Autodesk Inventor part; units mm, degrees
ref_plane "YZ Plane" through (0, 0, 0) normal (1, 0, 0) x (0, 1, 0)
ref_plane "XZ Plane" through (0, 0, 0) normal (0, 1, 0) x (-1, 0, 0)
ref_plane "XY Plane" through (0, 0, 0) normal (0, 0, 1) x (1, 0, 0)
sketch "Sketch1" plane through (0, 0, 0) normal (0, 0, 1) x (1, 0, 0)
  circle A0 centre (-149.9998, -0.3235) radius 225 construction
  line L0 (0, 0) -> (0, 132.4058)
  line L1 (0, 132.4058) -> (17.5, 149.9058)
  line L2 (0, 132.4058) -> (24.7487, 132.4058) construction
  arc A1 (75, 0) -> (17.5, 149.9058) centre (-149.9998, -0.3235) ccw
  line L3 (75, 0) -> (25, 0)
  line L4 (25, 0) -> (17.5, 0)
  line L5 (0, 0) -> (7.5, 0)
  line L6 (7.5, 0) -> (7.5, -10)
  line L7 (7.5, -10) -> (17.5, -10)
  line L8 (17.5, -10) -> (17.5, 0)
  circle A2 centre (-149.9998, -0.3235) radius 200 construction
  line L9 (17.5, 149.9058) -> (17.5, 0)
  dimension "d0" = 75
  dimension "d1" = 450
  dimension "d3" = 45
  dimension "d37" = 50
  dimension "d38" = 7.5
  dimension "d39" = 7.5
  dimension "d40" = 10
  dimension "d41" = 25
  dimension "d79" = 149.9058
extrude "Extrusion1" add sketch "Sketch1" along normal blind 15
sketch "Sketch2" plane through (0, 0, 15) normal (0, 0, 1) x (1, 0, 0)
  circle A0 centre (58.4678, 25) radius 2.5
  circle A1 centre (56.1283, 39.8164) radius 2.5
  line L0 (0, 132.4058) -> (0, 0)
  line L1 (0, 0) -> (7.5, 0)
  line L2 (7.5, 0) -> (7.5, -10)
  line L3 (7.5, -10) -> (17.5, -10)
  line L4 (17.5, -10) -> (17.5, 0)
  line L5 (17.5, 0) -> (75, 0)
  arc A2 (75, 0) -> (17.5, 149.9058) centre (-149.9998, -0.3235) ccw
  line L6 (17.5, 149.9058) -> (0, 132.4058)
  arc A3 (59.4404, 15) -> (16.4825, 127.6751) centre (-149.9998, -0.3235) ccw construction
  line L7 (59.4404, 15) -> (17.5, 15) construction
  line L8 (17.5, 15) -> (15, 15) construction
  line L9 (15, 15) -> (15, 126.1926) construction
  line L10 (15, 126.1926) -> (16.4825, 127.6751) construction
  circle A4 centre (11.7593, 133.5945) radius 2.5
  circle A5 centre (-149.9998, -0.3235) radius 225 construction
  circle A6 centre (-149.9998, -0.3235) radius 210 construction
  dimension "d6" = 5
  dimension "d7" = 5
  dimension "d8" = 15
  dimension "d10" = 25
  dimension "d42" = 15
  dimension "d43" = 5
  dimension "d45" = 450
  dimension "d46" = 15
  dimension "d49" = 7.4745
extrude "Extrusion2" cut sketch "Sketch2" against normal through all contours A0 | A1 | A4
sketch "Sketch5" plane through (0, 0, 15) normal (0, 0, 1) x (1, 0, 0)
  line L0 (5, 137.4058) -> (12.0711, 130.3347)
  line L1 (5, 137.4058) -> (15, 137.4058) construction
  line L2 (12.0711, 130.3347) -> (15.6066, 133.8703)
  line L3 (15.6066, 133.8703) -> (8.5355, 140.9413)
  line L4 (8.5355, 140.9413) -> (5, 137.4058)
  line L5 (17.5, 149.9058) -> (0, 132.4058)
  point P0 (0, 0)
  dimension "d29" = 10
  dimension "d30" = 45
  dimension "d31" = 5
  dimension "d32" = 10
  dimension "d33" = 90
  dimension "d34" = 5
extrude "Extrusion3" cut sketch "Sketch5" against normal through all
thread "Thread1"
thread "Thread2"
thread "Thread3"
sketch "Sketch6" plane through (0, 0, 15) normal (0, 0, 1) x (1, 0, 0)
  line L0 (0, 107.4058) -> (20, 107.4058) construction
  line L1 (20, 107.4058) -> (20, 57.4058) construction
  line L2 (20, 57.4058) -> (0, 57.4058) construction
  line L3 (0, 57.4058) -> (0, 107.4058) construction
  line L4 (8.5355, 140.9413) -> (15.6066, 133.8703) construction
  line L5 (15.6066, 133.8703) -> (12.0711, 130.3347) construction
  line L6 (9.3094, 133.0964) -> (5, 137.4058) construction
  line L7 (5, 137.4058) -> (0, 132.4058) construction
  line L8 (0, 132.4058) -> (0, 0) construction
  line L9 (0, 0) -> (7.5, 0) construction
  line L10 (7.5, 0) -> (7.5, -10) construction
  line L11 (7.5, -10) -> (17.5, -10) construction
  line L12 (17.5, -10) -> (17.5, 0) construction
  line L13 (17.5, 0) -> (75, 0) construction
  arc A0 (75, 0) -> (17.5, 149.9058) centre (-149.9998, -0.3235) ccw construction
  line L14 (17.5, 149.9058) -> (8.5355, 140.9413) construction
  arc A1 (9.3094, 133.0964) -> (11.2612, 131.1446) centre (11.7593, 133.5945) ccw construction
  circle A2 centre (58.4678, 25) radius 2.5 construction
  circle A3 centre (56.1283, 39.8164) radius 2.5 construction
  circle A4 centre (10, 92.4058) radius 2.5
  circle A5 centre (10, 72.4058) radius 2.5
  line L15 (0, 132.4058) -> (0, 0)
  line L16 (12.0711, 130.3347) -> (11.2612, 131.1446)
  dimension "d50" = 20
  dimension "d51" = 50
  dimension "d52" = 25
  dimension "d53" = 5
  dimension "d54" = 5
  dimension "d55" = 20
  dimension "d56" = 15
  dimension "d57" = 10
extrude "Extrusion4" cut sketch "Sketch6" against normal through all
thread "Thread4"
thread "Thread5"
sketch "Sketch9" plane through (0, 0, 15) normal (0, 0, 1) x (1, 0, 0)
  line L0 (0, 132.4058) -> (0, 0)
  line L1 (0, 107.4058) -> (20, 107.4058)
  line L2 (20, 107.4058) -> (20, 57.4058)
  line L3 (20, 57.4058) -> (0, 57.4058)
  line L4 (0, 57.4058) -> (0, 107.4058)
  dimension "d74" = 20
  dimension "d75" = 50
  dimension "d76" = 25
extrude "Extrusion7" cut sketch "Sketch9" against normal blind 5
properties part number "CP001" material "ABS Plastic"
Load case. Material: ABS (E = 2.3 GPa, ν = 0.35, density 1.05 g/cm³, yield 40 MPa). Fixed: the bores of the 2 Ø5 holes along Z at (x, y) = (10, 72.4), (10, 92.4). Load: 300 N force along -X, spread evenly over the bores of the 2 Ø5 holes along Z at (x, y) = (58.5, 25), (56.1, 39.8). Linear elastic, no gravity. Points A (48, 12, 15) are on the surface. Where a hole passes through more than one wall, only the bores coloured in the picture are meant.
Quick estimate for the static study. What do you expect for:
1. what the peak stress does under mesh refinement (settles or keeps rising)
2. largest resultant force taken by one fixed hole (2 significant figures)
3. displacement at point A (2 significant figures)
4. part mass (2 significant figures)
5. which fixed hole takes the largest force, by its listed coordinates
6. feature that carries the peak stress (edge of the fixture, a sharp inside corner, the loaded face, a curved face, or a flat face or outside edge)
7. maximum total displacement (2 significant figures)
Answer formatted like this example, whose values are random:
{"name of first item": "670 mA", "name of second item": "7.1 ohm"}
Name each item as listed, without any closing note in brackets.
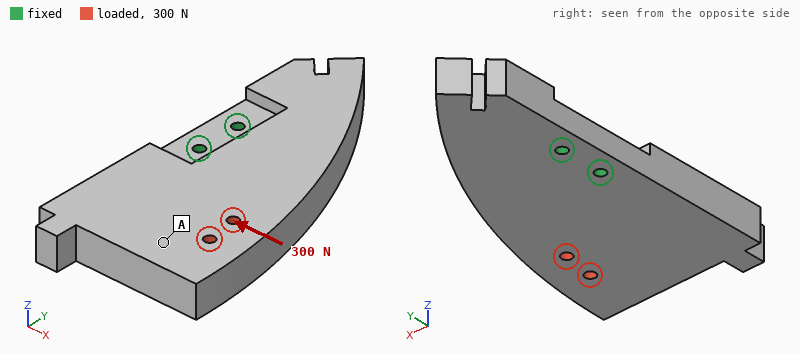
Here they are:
{"what the peak stress does under mesh refinement": "keeps rising", "largest resultant force taken by one fixed hole": "780 N", "displacement at point A": "0.25 mm", "part mass": "130 g", "which fixed hole takes the largest force, by its listed coordinates": "(10, 72.4)", "feature that carries the peak stress": "edge of the fixture", "maximum total displacement": "0.33 mm"}
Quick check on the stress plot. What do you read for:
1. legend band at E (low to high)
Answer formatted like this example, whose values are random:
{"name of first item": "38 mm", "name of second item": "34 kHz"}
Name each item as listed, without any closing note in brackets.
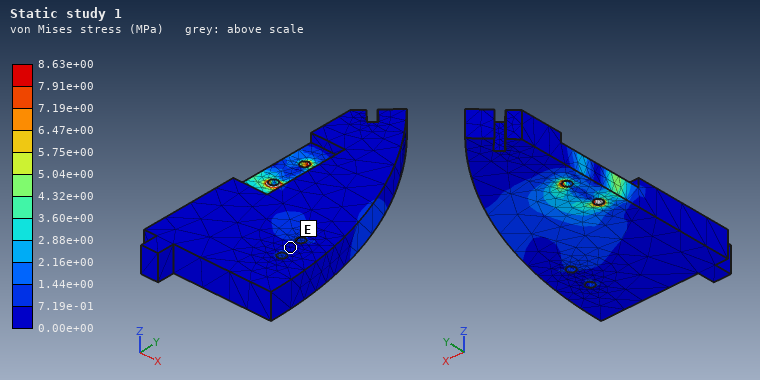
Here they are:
{"legend band at E": "0.00e+00 to 7.19e-01 MPa"}
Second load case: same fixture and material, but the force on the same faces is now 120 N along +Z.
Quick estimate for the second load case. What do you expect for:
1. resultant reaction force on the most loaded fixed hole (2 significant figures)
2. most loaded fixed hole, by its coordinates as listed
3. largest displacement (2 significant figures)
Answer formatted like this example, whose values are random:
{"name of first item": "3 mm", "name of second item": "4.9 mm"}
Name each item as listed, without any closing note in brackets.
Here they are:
{"resultant reaction force on the most loaded fixed hole": "230 N", "most loaded fixed hole, by its coordinates as listed": "(10, 72.4)", "largest displacement": "1.0 mm"}
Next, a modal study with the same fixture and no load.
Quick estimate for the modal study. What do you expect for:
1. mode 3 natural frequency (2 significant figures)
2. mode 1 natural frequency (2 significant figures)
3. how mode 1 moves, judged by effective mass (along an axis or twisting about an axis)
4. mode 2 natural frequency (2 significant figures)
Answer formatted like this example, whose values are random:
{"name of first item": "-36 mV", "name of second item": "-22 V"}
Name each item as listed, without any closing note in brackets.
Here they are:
{"mode 3 natural frequency": "620 Hz", "mode 1 natural frequency": "300 Hz", "how mode 1 moves, judged by effective mass": "along Z", "mode 2 natural frequency": "610 Hz"}
